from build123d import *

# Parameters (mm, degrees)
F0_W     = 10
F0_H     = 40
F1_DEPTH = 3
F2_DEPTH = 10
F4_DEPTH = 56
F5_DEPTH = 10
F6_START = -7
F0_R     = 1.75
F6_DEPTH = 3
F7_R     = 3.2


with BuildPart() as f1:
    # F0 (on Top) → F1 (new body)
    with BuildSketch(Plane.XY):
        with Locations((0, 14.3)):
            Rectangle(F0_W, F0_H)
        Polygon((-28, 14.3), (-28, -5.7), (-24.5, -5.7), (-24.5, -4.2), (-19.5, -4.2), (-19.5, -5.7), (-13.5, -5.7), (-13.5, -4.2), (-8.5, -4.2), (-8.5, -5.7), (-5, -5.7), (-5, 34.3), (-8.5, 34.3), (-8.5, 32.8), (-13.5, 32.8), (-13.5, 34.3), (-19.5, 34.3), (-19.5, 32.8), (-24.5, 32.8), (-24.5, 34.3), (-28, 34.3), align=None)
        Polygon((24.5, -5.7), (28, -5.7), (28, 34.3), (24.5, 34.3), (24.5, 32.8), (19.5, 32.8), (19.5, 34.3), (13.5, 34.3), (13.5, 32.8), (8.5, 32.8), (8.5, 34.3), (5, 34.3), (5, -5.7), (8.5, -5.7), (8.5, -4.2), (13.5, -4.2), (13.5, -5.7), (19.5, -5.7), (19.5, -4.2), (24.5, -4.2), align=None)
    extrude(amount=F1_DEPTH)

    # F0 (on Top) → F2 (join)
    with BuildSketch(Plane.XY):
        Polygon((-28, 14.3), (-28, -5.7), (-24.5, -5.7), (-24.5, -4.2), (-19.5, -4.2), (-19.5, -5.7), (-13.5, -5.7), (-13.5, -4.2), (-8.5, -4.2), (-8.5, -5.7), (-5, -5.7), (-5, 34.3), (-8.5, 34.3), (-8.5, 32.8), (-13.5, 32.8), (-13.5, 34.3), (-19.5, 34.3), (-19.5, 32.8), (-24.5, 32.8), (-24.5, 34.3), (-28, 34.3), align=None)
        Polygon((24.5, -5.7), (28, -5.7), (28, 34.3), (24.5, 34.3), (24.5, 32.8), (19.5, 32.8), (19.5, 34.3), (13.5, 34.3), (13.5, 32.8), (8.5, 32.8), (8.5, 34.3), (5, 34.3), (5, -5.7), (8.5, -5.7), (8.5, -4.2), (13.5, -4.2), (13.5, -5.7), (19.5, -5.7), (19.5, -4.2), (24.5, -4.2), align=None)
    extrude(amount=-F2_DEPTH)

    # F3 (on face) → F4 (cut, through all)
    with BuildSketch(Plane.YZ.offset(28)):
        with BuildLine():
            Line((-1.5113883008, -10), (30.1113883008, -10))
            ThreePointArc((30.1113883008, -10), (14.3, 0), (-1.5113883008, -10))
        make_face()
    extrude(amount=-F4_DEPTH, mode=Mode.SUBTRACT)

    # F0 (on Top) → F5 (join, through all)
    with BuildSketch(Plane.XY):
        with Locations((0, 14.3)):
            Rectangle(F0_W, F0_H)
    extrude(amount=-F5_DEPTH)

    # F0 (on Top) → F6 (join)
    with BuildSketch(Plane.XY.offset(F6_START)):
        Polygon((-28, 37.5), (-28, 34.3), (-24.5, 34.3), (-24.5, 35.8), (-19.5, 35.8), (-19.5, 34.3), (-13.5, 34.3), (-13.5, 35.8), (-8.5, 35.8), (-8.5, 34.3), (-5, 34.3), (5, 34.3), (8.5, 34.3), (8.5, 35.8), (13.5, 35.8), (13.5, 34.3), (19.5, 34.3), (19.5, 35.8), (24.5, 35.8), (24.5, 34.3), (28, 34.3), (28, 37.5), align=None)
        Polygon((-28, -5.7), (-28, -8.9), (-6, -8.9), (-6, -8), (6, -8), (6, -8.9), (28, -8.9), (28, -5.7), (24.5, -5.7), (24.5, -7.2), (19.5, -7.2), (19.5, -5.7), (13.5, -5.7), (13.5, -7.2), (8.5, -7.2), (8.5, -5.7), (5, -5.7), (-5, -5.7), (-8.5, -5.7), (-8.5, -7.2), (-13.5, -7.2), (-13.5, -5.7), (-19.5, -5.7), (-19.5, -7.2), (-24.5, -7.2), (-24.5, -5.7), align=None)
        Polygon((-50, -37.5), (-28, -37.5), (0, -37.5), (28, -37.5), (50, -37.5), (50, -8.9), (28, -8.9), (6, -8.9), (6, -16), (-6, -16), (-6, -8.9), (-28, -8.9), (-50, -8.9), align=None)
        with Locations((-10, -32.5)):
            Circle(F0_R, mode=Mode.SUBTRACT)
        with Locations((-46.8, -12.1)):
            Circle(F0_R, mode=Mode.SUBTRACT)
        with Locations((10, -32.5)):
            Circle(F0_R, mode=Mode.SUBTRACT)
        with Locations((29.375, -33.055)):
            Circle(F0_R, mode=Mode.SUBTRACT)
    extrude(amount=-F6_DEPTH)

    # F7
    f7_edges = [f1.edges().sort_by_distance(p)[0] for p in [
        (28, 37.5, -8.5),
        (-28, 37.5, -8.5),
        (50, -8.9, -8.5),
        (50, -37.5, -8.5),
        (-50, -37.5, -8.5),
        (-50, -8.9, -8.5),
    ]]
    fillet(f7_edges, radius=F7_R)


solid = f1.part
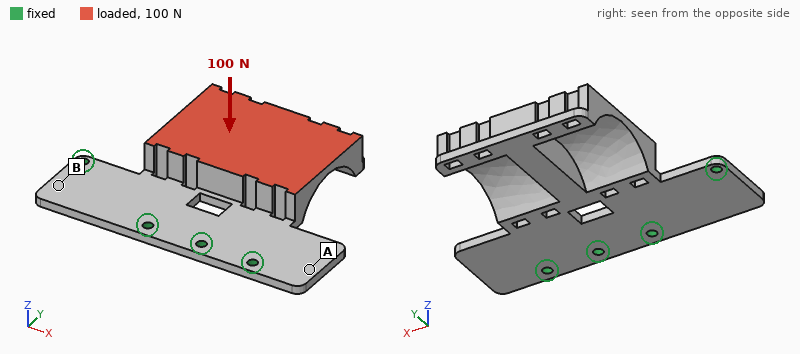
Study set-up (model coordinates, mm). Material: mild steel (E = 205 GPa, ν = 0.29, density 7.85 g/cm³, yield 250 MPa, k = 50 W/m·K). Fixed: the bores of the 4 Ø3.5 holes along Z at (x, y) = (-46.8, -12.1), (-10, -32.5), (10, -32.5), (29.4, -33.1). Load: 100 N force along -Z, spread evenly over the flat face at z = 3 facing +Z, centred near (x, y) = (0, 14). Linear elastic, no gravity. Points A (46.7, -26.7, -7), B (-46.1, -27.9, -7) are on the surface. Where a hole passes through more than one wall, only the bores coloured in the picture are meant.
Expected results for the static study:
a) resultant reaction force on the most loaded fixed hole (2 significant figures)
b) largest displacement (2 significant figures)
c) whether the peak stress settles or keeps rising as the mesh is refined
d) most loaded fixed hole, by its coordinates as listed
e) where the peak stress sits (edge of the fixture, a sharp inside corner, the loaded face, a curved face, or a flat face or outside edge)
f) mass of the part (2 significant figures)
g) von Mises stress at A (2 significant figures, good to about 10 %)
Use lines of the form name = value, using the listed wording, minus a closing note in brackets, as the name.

resultant reaction force on the most loaded fixed hole = 49 N
largest displacement = 0.17 mm
whether the peak stress settles or keeps rising as the mesh is refined = keeps rising
most loaded fixed hole, by its coordinates as listed = (-46.8, -12.1)
where the peak stress sits = edge of the fixture
mass of the part = 210 g
von Mises stress at A = 12 MPa
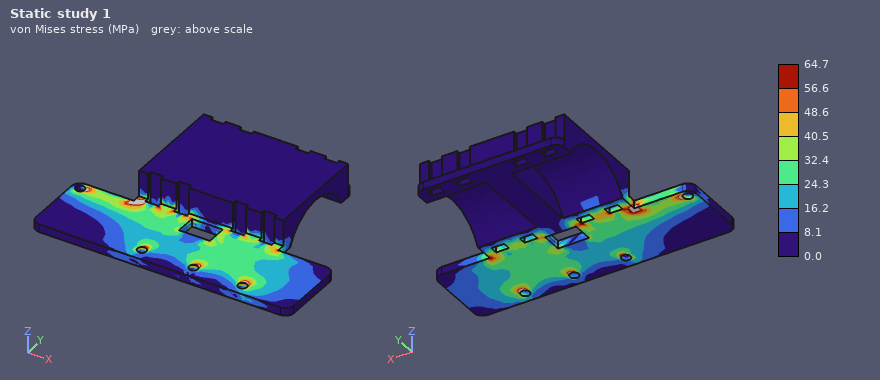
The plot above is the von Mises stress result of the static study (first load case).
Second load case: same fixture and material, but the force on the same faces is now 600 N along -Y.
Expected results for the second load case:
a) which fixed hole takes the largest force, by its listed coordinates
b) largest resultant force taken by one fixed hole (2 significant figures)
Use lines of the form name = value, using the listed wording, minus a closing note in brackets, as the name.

which fixed hole takes the largest force, by its listed coordinates = (-10, -32.5)
largest resultant force taken by one fixed hole = 280 N
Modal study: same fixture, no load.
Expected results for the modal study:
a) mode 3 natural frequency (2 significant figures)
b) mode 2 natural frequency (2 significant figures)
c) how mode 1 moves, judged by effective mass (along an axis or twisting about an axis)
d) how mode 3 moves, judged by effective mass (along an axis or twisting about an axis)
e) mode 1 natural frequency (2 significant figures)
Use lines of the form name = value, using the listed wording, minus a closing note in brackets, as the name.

mode 3 natural frequency = 3000 Hz
mode 2 natural frequency = 1900 Hz
how mode 1 moves, judged by effective mass = along Z
how mode 3 moves, judged by effective mass = along Z
mode 1 natural frequency = 380 Hz
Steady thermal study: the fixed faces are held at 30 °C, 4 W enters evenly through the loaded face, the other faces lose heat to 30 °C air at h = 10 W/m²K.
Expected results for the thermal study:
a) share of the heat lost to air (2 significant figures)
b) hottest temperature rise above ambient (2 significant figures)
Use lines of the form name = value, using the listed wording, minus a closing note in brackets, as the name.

share of the heat lost to air = 26 %
hottest temperature rise above ambient = 16 K
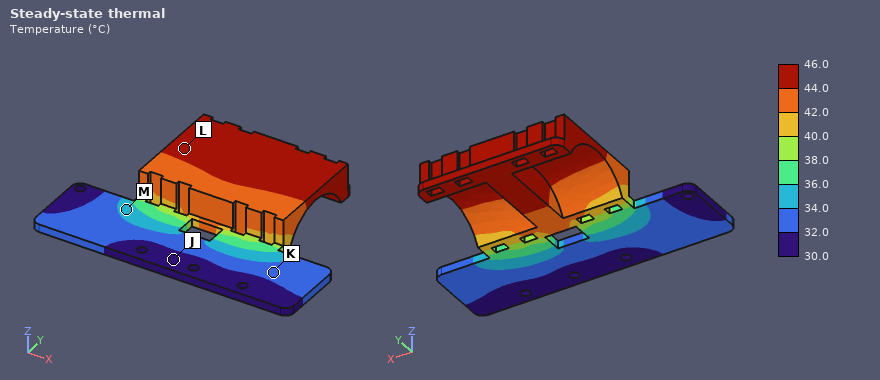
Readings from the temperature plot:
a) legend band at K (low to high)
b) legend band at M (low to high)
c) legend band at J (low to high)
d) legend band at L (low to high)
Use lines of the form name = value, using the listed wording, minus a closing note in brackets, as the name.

legend band at K = 32.0 to 34.0 °C
legend band at M = 34.0 to 36.0 °C
legend band at J = 30.0 to 32.0 °C
legend band at L = 44.0 to 46.0 °C
